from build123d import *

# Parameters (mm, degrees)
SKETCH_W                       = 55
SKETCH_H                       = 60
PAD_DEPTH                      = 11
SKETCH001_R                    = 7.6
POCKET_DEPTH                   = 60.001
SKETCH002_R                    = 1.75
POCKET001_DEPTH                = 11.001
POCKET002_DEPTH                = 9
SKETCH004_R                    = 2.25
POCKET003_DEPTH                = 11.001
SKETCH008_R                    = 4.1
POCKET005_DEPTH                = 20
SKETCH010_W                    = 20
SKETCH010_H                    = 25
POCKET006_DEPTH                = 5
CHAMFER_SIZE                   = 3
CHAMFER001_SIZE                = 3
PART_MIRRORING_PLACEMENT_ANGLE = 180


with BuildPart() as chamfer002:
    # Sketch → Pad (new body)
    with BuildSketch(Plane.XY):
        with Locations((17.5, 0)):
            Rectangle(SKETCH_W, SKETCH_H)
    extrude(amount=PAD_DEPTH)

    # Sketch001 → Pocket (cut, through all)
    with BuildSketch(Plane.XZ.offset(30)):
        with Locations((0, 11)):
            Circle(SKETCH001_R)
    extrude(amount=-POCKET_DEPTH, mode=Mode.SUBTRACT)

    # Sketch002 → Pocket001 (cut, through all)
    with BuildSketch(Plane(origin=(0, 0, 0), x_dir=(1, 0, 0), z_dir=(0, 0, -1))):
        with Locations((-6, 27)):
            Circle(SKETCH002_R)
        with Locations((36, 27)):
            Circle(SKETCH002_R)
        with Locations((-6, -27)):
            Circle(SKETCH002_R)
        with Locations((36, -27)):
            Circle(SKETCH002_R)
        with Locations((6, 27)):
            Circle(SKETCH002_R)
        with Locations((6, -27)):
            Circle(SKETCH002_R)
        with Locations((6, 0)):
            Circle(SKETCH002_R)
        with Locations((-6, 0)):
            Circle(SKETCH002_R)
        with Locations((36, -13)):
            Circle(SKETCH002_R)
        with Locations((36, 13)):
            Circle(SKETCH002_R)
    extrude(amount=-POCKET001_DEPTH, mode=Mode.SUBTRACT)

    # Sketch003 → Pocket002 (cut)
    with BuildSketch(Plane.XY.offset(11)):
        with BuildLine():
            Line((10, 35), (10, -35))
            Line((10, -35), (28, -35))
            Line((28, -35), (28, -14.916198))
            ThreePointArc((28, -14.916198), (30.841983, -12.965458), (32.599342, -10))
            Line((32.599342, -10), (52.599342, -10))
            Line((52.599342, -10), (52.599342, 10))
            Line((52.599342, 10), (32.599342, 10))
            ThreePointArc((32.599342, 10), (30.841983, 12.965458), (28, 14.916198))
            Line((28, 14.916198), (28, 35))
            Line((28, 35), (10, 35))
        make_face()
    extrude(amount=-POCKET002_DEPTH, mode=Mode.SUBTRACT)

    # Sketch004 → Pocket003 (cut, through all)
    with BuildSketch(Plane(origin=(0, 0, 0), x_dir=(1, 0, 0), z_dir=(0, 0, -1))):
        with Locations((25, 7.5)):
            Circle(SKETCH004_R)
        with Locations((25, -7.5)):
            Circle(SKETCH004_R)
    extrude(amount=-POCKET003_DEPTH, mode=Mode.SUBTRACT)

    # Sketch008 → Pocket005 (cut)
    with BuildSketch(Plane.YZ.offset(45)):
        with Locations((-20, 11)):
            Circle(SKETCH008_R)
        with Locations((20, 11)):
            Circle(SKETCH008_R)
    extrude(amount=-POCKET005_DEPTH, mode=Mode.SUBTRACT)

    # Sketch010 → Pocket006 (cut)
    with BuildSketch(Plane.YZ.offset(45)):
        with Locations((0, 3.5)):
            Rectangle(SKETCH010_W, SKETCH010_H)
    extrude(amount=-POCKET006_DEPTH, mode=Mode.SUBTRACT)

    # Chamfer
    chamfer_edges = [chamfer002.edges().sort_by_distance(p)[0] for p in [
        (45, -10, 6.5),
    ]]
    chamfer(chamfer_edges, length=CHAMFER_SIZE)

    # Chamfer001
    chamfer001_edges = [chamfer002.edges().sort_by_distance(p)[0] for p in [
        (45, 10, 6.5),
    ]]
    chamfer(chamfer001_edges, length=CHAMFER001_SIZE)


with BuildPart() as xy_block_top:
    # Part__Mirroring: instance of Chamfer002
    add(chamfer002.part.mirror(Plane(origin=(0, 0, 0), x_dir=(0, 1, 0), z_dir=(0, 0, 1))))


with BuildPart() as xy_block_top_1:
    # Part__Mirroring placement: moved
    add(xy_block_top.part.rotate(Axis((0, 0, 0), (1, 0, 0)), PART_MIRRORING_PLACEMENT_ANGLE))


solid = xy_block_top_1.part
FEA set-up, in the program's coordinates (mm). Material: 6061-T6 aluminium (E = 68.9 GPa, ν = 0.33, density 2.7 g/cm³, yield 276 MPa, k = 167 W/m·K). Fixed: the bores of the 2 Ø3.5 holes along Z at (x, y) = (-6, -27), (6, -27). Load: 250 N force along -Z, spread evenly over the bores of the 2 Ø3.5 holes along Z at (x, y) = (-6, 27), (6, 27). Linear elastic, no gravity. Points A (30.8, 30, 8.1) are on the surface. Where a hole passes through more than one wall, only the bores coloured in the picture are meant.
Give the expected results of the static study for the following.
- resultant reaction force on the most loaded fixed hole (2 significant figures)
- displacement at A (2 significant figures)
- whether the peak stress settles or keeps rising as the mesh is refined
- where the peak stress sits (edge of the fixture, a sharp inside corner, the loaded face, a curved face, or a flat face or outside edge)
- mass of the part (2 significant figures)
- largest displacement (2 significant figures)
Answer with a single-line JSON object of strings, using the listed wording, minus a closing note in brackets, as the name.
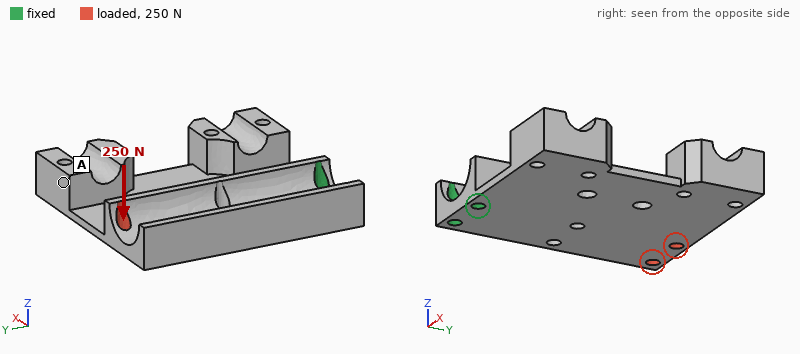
{"resultant reaction force on the most loaded fixed hole": "170 N", "displacement at A": "0.18 mm", "whether the peak stress settles or keeps rising as the mesh is refined": "keeps rising", "where the peak stress sits": "edge of the fixture", "mass of the part": "43 g", "largest displacement": "0.20 mm"}
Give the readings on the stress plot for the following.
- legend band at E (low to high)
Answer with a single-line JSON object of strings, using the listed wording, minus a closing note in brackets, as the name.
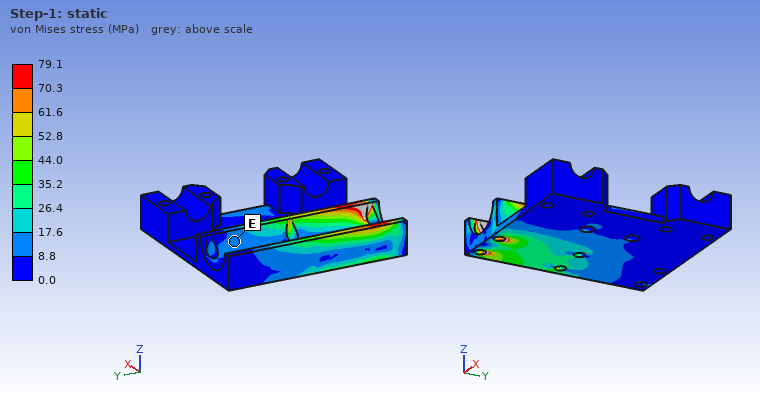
{"legend band at E": "8.8 to 17.6 MPa"}
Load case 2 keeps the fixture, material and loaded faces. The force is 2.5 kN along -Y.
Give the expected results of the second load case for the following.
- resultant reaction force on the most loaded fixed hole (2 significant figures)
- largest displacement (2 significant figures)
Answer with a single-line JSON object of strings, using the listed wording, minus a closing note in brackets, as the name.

{"resultant reaction force on the most loaded fixed hole": "1.3 kN", "largest displacement": "23 µm"}
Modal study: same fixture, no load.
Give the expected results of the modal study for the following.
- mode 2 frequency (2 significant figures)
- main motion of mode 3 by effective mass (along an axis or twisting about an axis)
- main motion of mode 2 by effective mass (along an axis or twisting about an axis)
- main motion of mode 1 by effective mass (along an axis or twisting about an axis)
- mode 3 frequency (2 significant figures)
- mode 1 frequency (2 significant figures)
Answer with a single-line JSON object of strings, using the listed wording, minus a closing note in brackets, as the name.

{"mode 2 frequency": "1100 Hz", "main motion of mode 3 by effective mass": "along Z", "main motion of mode 2 by effective mass": "twisting about X", "main motion of mode 1 by effective mass": "along Z", "mode 3 frequency": "2300 Hz", "mode 1 frequency": "640 Hz"}
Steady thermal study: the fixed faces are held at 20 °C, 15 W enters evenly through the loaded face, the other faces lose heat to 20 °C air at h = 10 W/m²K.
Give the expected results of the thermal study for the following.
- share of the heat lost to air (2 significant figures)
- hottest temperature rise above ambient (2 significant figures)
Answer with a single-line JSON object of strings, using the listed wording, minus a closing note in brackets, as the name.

{"share of the heat lost to air": "9.6 %", "hottest temperature rise above ambient": "32 K"}
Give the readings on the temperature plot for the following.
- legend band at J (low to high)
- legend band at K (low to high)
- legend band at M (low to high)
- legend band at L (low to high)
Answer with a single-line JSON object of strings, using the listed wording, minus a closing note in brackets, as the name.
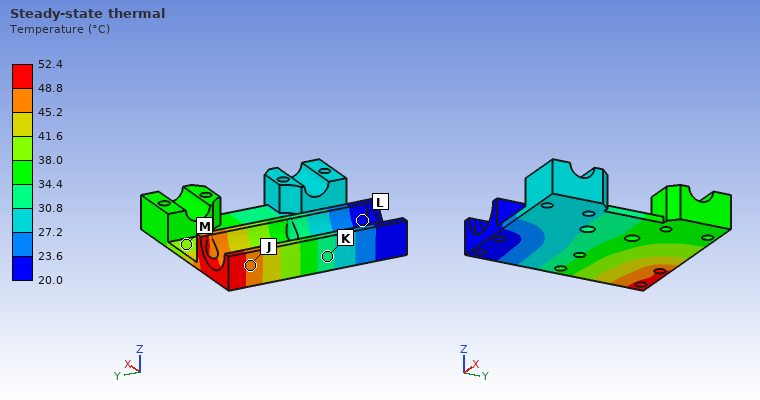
{"legend band at J": "45.2 to 48.8 °C", "legend band at K": "30.8 to 34.4 °C", "legend band at M": "38.0 to 41.6 °C", "legend band at L": "20.0 to 23.6 °C"}
